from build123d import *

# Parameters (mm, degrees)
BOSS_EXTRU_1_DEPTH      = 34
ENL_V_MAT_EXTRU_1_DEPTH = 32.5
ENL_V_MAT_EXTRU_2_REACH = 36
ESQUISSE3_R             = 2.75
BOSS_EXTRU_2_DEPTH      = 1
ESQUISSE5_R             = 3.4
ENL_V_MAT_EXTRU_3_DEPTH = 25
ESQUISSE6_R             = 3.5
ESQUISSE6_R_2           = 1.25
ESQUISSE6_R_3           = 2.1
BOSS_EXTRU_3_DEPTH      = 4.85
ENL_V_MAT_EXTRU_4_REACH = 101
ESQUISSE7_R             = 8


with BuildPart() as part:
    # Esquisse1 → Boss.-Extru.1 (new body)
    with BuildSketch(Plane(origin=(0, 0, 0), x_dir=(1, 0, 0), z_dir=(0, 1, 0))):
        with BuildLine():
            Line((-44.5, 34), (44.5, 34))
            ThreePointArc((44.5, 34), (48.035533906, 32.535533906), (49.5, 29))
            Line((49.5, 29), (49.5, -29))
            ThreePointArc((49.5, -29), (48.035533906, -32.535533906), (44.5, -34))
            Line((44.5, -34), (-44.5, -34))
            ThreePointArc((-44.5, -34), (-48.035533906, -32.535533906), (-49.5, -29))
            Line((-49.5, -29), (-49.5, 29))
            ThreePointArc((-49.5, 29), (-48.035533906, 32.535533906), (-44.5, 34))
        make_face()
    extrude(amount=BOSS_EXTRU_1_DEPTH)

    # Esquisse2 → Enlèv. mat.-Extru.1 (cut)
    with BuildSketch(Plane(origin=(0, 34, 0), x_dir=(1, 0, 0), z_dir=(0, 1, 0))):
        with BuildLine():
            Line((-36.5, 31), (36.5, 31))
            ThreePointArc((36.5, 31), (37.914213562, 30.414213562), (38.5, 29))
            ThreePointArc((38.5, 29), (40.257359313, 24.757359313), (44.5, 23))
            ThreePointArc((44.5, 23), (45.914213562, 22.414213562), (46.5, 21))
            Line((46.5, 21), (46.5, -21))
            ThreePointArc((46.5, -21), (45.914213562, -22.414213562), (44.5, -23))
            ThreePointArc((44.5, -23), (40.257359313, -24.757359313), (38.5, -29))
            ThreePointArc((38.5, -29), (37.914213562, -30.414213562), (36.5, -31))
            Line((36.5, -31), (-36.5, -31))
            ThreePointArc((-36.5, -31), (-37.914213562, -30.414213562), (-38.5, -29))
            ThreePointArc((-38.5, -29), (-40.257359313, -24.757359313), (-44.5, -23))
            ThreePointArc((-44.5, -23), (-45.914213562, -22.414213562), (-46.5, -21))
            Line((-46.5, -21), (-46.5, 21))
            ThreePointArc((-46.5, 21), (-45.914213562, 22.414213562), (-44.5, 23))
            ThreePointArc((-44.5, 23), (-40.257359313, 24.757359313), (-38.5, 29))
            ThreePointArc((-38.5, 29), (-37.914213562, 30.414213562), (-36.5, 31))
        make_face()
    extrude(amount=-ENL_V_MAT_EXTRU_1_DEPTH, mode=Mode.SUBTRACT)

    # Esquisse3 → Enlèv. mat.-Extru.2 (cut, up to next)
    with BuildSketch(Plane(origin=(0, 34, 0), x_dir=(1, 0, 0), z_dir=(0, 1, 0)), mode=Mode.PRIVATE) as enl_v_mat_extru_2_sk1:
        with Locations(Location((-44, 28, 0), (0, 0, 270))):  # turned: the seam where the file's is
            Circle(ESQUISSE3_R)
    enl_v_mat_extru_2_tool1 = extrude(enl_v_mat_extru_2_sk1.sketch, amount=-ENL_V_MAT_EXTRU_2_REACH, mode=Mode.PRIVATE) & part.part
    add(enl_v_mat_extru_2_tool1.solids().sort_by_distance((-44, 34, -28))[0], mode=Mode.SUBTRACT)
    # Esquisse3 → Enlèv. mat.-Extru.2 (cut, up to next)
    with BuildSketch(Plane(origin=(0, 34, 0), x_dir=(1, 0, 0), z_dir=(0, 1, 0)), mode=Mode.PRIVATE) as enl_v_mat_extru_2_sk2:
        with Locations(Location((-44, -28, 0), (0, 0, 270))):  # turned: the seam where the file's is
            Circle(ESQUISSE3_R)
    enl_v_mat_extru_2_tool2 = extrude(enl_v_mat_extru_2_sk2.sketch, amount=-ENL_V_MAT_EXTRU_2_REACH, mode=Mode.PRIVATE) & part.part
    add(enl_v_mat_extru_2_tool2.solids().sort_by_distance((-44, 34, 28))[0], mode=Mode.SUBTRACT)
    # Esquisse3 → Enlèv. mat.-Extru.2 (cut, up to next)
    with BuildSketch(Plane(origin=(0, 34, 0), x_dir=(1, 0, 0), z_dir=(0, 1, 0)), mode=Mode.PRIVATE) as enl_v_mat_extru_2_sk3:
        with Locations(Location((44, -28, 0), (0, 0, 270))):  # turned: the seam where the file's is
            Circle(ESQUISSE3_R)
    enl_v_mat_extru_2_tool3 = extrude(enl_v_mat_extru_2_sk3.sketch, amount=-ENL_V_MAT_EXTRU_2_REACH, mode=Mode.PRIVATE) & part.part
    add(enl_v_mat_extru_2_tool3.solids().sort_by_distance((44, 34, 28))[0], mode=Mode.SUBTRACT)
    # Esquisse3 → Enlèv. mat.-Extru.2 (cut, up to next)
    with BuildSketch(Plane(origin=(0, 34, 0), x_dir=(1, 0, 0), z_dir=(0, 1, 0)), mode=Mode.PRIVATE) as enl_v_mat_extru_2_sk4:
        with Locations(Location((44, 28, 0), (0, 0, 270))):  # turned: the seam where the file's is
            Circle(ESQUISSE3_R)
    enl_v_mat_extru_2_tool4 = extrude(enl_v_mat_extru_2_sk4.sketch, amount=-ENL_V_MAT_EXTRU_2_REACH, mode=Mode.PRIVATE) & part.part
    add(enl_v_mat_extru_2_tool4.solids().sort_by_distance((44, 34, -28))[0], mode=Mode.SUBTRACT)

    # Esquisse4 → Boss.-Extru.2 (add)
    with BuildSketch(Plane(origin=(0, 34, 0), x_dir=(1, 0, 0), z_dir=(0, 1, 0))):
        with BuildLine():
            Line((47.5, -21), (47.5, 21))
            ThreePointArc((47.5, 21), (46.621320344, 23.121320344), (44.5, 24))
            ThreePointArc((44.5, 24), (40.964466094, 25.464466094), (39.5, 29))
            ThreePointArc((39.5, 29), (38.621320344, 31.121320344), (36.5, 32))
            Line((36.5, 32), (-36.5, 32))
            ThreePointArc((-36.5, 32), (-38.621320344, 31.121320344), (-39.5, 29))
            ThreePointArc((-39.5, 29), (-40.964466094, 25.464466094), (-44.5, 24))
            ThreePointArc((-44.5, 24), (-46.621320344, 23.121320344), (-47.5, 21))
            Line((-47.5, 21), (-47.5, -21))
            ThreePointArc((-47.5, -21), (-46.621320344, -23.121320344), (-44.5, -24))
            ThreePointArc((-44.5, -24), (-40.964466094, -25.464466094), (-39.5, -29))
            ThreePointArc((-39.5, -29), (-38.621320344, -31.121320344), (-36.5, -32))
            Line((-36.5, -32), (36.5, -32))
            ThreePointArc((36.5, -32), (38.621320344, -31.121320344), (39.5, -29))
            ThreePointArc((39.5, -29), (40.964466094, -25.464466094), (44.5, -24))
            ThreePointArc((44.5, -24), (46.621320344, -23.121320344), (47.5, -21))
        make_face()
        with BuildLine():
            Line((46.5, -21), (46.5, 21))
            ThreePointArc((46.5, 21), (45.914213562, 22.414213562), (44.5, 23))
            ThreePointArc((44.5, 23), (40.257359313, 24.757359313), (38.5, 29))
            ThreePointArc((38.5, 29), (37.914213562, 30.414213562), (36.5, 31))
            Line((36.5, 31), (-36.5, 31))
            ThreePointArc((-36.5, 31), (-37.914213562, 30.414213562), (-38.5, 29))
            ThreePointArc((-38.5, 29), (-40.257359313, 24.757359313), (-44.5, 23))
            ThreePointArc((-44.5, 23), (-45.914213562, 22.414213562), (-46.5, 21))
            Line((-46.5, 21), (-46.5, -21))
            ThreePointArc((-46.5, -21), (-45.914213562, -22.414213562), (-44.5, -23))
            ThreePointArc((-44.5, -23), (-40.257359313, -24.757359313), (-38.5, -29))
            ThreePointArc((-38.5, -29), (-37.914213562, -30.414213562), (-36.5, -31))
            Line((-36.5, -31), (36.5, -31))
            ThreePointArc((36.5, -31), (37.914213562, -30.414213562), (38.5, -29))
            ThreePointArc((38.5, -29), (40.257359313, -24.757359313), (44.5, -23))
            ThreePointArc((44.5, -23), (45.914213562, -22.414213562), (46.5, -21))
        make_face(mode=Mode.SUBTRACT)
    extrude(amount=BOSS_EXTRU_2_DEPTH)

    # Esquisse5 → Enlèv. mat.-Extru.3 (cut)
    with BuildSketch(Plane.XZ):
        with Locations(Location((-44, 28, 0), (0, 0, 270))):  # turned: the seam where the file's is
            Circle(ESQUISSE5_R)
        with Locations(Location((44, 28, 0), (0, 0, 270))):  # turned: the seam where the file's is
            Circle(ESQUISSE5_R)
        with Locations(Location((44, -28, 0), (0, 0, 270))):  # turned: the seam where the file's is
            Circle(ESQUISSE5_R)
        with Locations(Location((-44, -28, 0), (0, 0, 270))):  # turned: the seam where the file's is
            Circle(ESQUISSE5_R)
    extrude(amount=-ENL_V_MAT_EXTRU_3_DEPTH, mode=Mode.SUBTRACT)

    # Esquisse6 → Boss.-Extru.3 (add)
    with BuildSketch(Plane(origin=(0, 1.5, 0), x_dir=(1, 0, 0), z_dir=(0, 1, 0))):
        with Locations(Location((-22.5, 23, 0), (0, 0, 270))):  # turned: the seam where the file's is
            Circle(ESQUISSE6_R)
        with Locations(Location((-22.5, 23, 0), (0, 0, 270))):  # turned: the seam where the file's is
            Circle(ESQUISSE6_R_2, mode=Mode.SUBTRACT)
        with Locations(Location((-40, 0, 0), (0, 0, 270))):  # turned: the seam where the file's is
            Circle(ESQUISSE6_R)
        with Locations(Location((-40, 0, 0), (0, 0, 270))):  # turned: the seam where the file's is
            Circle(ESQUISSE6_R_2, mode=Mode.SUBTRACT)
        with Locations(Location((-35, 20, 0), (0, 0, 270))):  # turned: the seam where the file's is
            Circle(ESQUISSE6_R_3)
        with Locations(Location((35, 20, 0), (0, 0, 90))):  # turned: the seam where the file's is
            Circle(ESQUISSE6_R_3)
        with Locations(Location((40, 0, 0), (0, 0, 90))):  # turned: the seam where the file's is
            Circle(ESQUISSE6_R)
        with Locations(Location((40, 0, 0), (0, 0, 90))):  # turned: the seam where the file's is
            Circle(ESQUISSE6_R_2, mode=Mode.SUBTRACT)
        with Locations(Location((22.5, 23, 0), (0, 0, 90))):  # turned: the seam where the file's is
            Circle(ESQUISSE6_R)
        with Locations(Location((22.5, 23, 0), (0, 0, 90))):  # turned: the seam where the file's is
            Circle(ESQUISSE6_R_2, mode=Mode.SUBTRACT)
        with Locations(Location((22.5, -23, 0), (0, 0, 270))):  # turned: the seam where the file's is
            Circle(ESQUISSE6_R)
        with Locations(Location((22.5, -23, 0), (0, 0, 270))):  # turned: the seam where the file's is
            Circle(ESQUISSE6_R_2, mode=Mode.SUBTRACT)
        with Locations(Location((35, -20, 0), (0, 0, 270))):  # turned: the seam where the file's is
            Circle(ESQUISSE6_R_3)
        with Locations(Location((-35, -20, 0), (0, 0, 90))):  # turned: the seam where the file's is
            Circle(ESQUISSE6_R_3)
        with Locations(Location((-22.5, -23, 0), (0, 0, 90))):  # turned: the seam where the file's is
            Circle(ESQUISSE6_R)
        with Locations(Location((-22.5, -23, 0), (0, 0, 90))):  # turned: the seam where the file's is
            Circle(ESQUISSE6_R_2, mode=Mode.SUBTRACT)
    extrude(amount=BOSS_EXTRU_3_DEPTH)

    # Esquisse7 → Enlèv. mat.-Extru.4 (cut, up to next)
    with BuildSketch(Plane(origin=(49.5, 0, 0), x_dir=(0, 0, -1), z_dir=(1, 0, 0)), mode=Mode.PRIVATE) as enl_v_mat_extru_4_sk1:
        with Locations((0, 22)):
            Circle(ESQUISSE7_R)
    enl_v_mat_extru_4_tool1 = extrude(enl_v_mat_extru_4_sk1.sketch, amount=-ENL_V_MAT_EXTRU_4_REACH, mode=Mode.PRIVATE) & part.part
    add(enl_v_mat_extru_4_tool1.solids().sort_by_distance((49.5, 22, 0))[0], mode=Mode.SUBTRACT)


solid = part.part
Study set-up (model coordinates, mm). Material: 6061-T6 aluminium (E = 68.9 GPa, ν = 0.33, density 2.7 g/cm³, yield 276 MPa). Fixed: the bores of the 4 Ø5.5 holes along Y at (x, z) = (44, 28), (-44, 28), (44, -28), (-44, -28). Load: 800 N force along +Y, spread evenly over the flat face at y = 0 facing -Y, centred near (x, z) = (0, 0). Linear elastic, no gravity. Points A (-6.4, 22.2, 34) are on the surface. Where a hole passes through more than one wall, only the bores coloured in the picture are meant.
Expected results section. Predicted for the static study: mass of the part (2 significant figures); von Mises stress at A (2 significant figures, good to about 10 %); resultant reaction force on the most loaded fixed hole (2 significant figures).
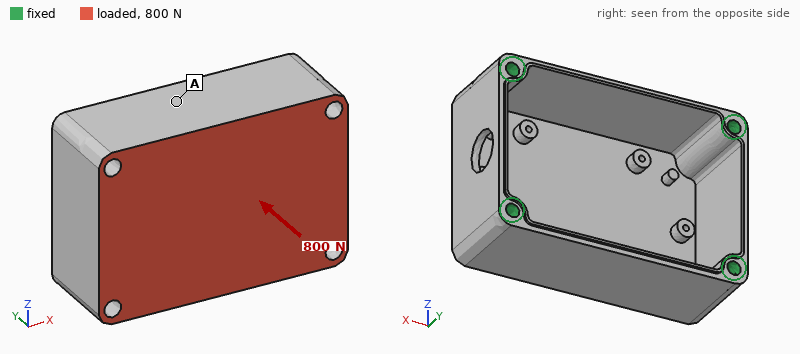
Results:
120 g
6.7 MPa
220 N
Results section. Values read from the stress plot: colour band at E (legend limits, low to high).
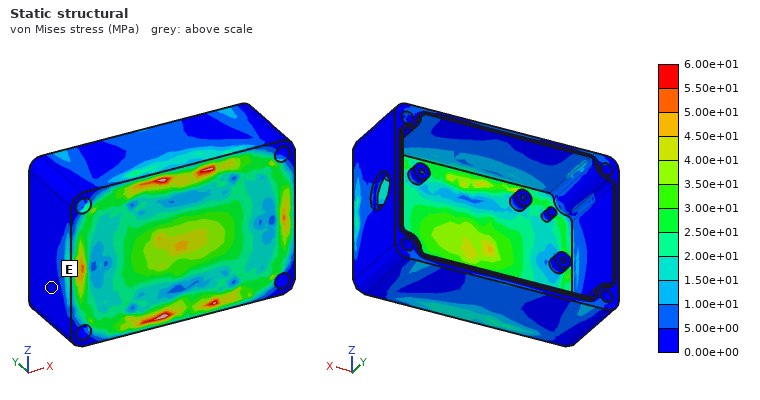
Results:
0.00e+00 to 5.00e+00 MPa
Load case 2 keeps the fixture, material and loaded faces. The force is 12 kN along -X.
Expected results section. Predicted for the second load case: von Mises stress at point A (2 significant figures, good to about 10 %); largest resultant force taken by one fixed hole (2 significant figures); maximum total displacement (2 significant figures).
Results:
30 MPa
3.5 kN
66 µm
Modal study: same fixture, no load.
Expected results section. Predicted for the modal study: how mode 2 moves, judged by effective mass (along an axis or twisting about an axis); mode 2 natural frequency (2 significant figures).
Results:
along Z
3200 Hz
